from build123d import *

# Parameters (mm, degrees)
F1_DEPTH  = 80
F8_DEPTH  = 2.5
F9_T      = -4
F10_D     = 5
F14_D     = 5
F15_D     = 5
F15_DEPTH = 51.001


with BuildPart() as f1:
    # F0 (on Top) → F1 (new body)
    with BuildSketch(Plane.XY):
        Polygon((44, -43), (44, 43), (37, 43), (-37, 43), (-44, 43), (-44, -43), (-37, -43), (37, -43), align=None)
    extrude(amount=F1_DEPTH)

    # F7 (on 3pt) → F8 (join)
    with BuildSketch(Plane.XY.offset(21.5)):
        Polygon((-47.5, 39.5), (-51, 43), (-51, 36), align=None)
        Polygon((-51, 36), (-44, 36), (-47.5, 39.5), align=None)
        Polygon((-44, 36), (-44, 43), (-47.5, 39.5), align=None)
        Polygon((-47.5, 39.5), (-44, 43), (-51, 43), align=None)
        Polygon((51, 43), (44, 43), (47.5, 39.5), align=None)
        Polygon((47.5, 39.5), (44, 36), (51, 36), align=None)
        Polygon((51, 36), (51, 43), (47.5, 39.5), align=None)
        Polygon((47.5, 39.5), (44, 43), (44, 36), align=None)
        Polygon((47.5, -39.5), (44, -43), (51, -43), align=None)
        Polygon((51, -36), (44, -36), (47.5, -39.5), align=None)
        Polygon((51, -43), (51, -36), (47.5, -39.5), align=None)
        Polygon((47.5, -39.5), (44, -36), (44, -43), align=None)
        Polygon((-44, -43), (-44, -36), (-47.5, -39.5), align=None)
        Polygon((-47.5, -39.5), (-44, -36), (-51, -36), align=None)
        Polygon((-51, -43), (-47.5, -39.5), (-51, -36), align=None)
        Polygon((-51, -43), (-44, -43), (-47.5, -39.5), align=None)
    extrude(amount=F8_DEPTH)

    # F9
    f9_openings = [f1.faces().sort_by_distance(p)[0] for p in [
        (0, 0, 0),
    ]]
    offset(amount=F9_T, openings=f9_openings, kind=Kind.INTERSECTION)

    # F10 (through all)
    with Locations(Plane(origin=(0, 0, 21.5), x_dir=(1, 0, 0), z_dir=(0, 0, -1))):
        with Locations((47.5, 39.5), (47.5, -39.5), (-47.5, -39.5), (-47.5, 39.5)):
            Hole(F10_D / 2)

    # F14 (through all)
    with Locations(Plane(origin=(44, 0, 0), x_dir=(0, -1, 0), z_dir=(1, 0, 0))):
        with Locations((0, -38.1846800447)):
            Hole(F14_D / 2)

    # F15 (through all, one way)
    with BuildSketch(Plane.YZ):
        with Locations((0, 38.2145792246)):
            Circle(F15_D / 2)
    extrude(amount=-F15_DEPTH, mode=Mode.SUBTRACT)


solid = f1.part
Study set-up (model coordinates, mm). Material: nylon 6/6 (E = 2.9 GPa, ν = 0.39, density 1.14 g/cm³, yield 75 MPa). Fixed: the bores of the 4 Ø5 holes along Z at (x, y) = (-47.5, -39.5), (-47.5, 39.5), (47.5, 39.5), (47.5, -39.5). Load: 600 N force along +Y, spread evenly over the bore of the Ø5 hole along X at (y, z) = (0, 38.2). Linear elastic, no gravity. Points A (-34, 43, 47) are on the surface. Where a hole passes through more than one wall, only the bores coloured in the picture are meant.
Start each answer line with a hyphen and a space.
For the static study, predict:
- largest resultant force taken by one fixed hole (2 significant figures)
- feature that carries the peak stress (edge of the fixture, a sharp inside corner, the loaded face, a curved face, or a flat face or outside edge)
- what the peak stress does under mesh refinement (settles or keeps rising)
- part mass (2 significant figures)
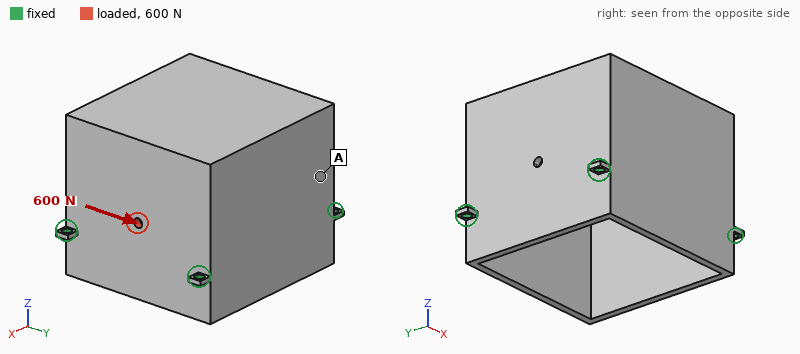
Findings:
- 280 N
- edge of the fixture
- keeps rising
- 150 g
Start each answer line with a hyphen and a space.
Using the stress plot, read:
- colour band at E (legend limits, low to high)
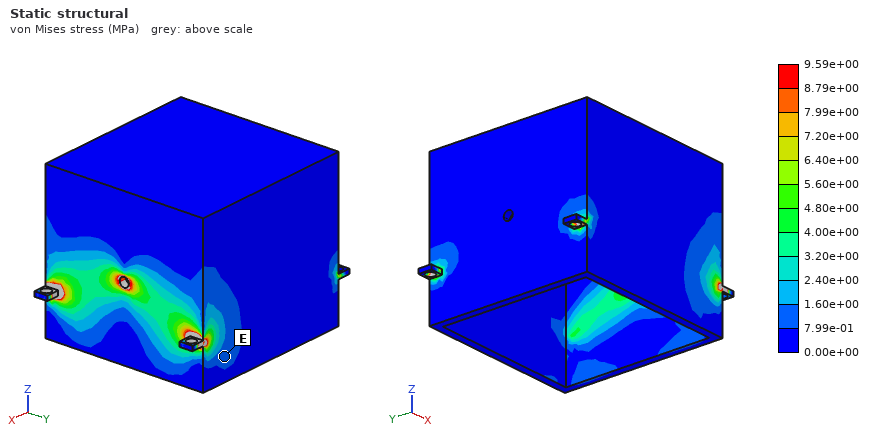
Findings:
- 7.99e-01 to 1.60e+00 MPa
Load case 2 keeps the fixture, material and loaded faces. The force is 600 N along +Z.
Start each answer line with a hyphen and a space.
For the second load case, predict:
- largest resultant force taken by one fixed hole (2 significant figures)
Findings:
- 290 N
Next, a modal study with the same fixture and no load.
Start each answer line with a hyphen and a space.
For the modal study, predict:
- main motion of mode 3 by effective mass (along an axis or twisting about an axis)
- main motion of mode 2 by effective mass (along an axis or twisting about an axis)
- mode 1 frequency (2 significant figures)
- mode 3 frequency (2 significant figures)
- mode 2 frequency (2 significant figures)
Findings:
- along X
- along Y
- 720 Hz
- 940 Hz
- 770 Hz
